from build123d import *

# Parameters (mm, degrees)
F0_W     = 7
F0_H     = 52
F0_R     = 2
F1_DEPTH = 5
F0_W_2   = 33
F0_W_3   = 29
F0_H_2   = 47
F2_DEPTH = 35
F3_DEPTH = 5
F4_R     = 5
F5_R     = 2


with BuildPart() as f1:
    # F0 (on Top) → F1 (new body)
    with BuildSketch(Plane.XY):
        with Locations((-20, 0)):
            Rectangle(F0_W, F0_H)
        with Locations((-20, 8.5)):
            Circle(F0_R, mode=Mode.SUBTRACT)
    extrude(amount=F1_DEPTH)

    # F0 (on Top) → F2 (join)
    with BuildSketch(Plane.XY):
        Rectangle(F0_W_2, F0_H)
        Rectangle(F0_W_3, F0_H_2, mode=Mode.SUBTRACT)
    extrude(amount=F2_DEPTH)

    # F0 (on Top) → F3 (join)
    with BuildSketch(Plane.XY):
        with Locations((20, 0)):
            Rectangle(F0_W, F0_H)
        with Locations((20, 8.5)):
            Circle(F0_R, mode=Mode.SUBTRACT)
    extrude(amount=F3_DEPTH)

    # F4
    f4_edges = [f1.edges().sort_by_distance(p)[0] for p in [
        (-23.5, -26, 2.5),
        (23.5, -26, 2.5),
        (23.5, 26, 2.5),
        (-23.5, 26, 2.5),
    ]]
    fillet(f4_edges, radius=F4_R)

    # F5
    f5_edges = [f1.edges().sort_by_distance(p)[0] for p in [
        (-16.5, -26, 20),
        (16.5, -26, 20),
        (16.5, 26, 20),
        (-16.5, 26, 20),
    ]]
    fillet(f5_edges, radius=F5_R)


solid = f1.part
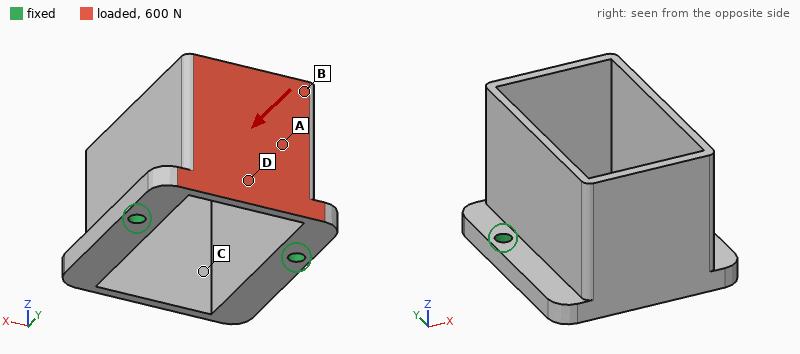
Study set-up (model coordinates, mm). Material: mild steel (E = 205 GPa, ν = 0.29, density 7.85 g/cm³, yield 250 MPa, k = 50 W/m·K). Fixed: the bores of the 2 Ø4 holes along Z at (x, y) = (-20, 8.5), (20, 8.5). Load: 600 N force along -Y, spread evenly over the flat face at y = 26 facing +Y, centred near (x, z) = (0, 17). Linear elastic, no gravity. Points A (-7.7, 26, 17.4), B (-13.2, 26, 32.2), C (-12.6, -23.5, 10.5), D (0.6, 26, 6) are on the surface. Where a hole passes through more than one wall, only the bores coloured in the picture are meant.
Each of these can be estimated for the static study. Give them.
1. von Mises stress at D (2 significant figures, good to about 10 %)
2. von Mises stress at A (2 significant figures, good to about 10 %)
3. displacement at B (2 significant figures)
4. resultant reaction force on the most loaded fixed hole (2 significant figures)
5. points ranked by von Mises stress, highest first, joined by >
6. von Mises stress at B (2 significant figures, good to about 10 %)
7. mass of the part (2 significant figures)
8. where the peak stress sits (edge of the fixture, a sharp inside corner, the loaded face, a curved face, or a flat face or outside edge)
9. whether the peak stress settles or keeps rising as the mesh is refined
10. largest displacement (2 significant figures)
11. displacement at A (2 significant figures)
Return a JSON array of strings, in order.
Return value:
["32 MPa", "19 MPa", "19 µm", "320 N", "D > A > B > C", "10 MPa", "120 g", "edge of the fixture", "keeps rising", "32 µm", "17 µm"]
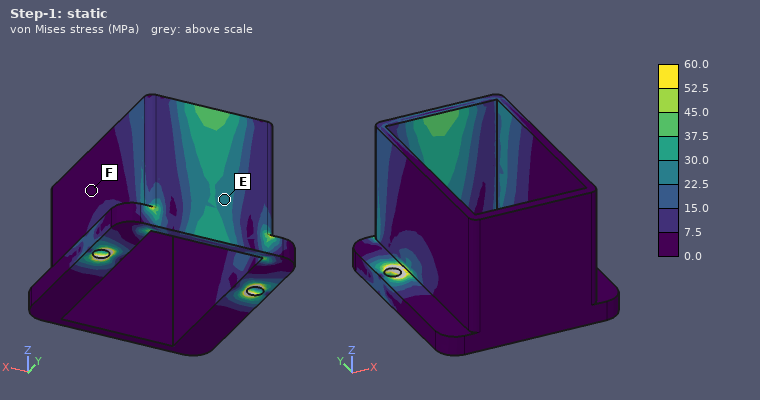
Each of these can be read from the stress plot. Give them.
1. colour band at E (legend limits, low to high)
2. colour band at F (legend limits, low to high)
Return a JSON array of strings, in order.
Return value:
["22.5 to 30.0 MPa", "0.0 to 7.5 MPa"]
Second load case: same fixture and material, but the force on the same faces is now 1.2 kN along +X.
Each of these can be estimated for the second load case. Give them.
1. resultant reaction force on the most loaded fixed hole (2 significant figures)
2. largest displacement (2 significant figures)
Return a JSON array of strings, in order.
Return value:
["790 N", "28 µm"]
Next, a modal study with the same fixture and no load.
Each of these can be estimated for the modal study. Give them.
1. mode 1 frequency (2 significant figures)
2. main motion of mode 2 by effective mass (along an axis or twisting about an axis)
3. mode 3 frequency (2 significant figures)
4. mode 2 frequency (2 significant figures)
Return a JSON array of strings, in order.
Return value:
["2400 Hz", "along X", "4200 Hz", "2700 Hz"]
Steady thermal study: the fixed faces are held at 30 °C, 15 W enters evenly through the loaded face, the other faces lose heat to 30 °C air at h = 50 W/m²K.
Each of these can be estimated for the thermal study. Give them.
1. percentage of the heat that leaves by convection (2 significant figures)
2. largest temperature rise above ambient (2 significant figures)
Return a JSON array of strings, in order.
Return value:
["43 %", "41 K"]
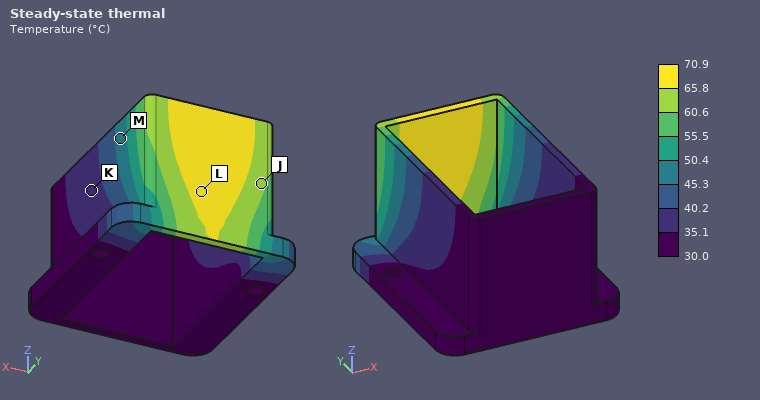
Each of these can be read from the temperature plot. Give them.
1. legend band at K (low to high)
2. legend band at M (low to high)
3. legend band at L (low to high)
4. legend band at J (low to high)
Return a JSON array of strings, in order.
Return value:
["35.1 to 40.2 °C", "45.3 to 50.4 °C", "65.8 to 70.9 °C", "60.6 to 65.8 °C"]
